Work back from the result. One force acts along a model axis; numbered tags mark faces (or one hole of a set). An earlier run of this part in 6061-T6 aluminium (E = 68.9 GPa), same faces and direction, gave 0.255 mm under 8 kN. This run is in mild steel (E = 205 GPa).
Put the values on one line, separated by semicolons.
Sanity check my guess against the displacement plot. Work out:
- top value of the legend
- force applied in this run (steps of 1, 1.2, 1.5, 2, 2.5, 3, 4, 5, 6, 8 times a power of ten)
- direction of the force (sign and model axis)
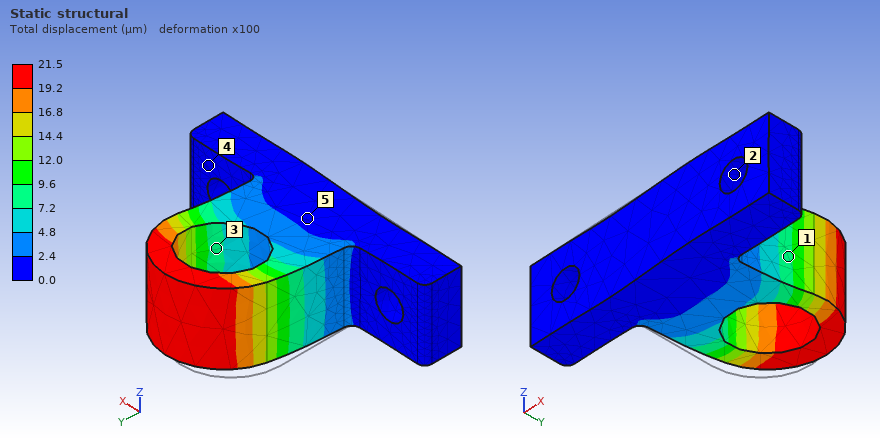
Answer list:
21.5 µm; 2 kN; +X
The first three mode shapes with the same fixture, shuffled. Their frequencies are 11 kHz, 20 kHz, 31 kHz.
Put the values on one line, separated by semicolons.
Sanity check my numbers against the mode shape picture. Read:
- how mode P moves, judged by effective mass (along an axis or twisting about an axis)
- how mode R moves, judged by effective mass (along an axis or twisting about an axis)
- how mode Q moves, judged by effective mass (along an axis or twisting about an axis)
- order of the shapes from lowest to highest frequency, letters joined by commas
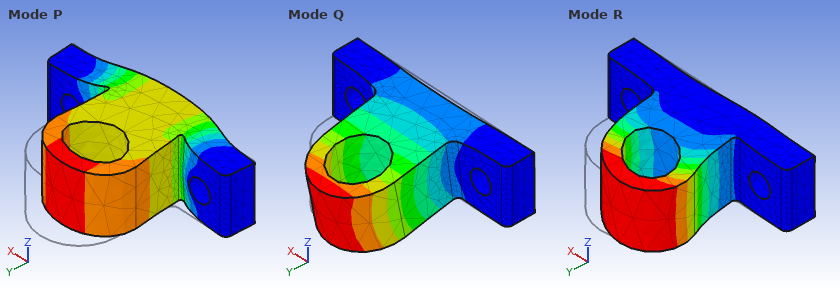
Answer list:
along Y; along X; along Z; Q, R, P
